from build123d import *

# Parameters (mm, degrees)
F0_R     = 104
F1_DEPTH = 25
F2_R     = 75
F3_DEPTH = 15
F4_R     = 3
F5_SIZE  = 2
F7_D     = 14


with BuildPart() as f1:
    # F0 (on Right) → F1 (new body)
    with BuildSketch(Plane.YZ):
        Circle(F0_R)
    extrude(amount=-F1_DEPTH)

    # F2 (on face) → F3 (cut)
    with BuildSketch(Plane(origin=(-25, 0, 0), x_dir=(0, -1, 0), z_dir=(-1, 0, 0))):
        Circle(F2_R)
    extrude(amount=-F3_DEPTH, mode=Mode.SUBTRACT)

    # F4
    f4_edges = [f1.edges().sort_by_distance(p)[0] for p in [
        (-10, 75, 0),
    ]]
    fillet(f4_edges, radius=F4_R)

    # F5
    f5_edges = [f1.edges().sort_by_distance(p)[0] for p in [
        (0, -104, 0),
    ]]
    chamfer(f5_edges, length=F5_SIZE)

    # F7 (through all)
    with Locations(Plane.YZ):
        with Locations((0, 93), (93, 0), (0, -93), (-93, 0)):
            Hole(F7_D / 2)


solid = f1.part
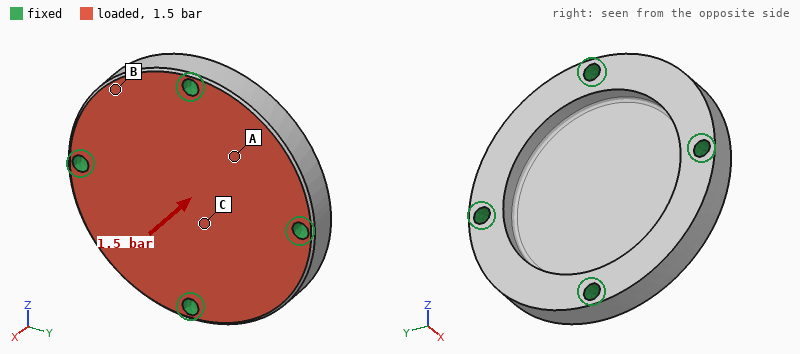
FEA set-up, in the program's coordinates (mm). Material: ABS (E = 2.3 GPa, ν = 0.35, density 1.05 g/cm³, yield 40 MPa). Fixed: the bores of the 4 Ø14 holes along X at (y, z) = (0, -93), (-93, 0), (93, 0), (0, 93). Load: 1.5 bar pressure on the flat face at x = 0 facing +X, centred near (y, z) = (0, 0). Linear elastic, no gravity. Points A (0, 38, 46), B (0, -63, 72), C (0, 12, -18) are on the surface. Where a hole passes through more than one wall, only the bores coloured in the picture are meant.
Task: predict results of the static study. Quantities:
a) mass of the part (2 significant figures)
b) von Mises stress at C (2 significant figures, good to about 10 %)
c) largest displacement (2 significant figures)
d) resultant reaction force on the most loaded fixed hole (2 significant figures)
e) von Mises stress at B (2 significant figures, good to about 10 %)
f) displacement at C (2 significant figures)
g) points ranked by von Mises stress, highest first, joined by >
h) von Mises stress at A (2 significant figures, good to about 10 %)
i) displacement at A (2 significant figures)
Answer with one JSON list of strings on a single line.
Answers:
["600 g", "4.6 MPa", "0.56 mm", "1.2 kN", "1.5 MPa", "0.50 mm", "C > A > B", "3.0 MPa", "0.20 mm"]
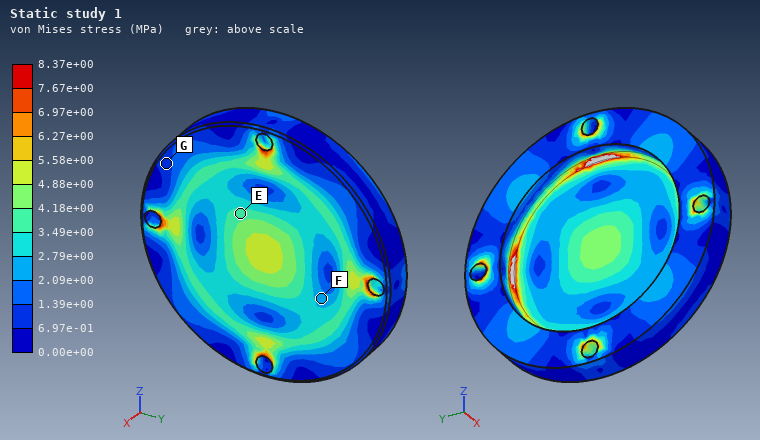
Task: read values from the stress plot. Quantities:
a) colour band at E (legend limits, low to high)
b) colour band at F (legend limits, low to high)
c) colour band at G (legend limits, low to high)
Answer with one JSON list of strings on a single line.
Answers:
["3.49e+00 to 4.18e+00 MPa", "2.09e+00 to 2.79e+00 MPa", "6.97e-01 to 1.39e+00 MPa"]
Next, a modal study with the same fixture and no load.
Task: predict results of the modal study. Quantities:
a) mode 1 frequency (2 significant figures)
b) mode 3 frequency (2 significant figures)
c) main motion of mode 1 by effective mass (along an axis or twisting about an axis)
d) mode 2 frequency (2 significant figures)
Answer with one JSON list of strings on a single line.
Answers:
["1000 Hz", "1600 Hz", "along X", "1600 Hz"]
